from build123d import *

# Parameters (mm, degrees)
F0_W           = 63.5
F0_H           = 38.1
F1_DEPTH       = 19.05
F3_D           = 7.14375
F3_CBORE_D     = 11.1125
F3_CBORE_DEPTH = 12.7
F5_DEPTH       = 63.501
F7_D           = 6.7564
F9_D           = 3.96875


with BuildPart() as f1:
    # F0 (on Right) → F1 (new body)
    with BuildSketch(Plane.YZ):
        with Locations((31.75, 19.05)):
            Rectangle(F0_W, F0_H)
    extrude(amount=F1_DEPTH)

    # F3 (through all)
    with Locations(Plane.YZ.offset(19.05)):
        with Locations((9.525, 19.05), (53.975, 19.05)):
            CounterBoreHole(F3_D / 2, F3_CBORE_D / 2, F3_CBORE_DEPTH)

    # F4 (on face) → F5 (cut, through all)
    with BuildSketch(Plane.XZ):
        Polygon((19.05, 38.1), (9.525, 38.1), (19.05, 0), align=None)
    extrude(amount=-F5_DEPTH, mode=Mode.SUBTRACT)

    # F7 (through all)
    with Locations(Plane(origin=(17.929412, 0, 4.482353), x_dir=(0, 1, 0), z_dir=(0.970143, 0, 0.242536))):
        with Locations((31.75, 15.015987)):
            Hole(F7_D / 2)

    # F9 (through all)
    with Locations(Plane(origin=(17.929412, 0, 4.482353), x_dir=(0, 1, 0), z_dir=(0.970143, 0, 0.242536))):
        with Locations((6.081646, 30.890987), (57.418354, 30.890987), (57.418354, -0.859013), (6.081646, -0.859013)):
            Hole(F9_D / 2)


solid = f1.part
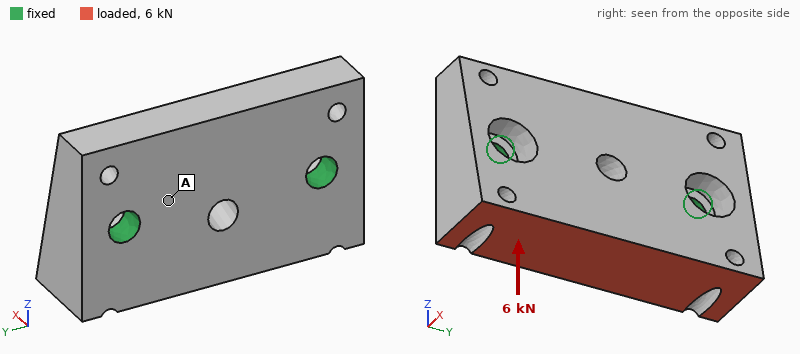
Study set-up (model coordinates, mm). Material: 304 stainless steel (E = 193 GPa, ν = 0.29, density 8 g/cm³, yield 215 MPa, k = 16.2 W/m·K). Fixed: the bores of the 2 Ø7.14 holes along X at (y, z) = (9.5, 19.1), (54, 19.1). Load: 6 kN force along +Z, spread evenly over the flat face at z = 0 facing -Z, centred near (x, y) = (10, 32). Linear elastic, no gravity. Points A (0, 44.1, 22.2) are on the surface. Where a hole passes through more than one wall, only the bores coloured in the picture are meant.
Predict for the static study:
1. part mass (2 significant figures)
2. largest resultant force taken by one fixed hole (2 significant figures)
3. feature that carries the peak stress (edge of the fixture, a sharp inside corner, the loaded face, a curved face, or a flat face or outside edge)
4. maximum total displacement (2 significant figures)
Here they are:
250 g
3.0 kN
the loaded face
12 µm
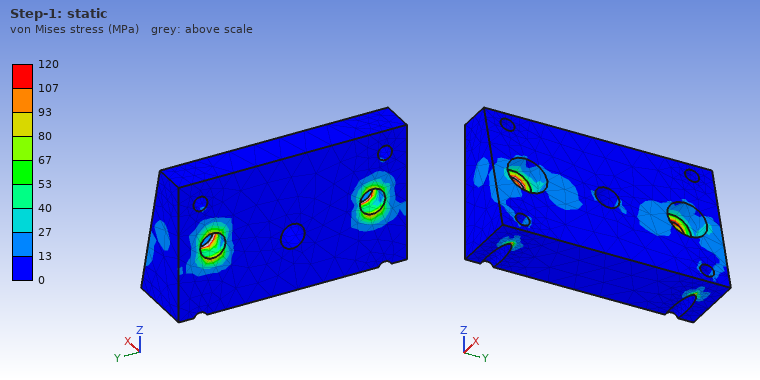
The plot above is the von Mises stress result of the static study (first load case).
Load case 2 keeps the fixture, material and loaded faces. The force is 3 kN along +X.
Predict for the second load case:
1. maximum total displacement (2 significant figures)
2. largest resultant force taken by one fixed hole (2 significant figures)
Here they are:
17 µm
1.6 kN
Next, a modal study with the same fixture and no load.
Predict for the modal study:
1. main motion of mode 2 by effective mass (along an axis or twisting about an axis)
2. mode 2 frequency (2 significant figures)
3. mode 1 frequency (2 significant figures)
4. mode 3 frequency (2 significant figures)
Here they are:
along X
15 kHz
8000 Hz
16 kHz
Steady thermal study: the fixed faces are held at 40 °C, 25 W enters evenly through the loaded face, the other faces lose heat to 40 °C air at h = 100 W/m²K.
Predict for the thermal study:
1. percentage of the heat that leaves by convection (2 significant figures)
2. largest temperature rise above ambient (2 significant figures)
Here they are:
43 %
39 K
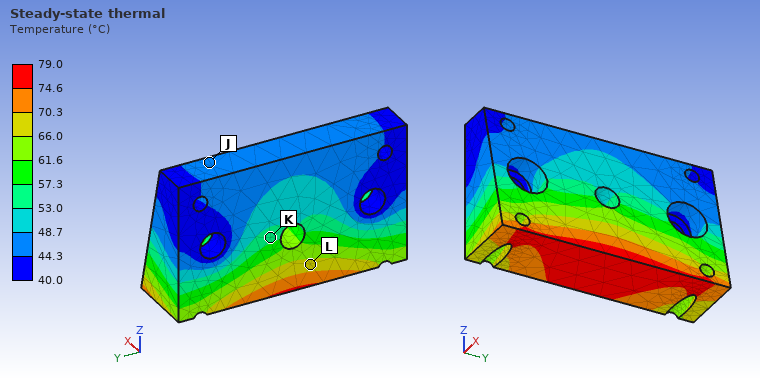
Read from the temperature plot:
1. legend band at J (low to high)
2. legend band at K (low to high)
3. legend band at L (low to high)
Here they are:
44.3 to 48.7 °C
53.0 to 57.3 °C
66.0 to 70.3 °C
